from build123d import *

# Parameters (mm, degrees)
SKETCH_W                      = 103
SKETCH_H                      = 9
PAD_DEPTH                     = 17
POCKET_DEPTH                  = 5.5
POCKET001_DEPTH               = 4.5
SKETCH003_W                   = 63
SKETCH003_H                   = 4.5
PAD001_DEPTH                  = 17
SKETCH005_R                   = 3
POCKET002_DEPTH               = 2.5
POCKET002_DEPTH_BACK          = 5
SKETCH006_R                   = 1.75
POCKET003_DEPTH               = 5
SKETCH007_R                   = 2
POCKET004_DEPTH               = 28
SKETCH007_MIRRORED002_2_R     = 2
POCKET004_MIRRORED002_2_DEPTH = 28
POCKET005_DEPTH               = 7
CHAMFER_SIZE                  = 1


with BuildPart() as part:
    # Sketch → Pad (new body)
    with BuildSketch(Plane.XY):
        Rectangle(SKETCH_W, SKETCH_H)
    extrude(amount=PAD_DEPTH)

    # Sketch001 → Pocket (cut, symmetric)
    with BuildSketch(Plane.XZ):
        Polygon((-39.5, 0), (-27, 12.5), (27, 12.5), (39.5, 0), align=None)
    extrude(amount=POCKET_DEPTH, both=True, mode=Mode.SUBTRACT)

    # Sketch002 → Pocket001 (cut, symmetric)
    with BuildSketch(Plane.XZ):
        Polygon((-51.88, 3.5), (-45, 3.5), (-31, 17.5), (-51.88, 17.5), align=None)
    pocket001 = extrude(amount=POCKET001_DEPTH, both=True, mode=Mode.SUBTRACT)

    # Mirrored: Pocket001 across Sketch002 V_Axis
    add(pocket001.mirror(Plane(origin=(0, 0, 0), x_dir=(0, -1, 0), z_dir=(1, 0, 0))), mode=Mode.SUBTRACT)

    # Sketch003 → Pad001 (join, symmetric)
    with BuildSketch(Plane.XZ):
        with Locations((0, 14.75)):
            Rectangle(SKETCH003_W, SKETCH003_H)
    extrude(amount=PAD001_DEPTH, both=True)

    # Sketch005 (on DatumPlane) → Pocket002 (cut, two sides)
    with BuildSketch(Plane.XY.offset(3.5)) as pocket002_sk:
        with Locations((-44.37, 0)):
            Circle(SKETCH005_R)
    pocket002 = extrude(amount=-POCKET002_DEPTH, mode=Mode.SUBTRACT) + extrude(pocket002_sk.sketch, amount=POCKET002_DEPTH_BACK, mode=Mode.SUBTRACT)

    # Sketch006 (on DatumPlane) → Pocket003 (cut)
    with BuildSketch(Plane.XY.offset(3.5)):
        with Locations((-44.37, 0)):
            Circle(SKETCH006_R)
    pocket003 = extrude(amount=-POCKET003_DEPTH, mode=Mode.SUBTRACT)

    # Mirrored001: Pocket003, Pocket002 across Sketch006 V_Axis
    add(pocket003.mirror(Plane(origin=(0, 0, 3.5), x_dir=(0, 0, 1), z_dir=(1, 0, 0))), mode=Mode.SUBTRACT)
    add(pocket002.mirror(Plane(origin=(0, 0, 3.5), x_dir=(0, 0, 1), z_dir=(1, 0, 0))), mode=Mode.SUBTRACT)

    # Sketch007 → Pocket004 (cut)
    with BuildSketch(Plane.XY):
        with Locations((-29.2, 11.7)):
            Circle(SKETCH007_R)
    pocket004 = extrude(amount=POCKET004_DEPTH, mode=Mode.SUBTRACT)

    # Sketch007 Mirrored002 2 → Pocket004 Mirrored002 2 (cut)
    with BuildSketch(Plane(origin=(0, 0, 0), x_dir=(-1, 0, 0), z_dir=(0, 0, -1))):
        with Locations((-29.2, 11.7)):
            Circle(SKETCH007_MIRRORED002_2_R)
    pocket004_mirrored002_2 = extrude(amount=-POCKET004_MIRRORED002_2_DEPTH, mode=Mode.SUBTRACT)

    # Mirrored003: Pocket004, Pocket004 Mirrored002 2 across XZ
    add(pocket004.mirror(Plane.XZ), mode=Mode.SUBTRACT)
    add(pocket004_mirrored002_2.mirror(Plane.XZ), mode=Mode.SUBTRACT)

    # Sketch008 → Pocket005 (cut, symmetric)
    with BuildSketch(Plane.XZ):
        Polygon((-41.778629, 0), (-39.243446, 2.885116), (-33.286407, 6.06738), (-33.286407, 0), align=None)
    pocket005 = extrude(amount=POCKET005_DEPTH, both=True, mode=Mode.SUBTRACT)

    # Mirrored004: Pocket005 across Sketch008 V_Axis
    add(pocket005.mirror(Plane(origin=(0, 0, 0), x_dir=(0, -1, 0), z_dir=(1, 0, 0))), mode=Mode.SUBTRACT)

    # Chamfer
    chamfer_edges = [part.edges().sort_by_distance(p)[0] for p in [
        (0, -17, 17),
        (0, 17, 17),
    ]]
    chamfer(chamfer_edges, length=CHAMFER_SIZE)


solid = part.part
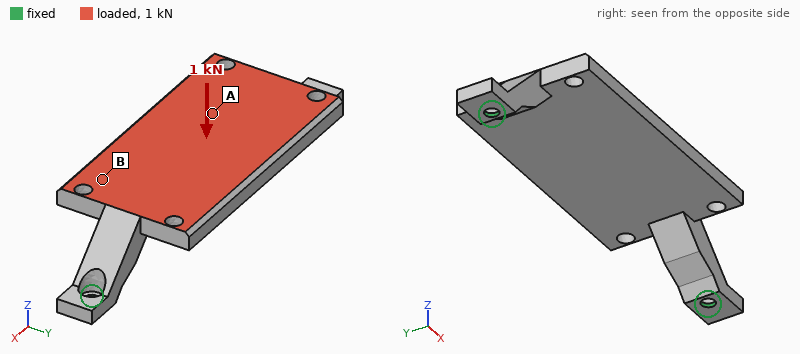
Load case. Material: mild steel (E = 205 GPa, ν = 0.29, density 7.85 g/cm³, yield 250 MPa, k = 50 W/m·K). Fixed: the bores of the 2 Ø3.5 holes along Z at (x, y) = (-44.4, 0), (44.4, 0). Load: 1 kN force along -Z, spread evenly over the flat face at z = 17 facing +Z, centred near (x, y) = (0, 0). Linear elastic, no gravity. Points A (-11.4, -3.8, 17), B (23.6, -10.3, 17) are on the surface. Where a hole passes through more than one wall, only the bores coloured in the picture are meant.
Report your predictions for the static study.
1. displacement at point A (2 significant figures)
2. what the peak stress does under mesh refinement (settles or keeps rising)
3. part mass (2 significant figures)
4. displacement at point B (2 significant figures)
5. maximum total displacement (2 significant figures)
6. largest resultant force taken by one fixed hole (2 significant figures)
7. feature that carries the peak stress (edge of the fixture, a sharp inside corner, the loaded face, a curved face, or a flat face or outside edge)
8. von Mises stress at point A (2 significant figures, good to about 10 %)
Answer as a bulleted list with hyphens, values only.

- 26 µm
- keeps rising
- 90 g
- 15 µm
- 33 µm
- 880 N
- edge of the fixture
- 33 MPa
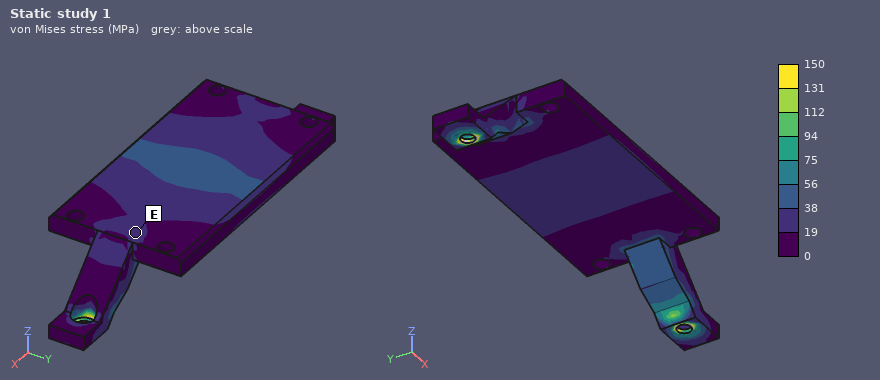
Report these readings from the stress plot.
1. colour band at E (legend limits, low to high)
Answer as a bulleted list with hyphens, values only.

- 19 to 38 MPa
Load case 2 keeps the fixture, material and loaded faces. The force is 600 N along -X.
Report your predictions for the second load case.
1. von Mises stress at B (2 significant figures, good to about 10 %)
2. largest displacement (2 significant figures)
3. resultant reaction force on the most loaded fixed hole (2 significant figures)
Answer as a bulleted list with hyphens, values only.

- 13 MPa
- 15 µm
- 320 N
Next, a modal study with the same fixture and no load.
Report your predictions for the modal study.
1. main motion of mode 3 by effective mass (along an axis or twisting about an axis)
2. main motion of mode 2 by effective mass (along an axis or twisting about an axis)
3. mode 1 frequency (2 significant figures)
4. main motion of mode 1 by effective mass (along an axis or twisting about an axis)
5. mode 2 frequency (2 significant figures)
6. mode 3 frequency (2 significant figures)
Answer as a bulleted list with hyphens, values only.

- along Z
- along X
- 1300 Hz
- along Y
- 3300 Hz
- 3700 Hz
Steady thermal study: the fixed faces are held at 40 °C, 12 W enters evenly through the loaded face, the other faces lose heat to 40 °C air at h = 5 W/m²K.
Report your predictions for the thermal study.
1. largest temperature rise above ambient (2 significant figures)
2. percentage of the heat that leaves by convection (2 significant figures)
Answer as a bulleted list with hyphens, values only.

- 76 K
- 11 %
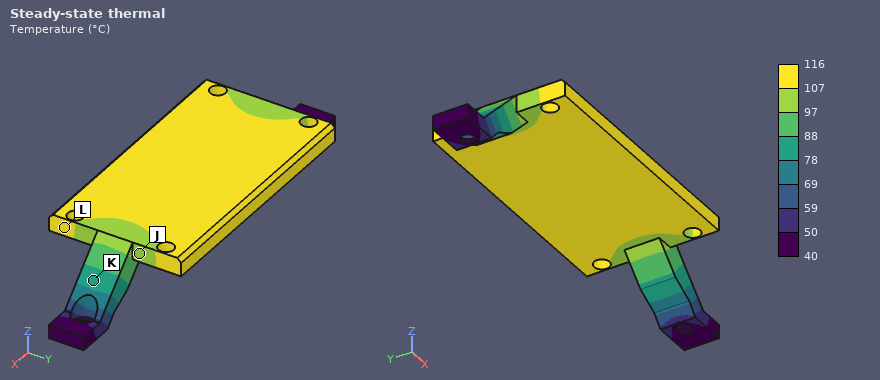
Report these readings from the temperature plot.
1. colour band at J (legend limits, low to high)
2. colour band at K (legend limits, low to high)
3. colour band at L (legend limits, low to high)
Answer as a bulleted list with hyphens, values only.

- 97 to 107 °C
- 78 to 88 °C
- 107 to 116 °C
